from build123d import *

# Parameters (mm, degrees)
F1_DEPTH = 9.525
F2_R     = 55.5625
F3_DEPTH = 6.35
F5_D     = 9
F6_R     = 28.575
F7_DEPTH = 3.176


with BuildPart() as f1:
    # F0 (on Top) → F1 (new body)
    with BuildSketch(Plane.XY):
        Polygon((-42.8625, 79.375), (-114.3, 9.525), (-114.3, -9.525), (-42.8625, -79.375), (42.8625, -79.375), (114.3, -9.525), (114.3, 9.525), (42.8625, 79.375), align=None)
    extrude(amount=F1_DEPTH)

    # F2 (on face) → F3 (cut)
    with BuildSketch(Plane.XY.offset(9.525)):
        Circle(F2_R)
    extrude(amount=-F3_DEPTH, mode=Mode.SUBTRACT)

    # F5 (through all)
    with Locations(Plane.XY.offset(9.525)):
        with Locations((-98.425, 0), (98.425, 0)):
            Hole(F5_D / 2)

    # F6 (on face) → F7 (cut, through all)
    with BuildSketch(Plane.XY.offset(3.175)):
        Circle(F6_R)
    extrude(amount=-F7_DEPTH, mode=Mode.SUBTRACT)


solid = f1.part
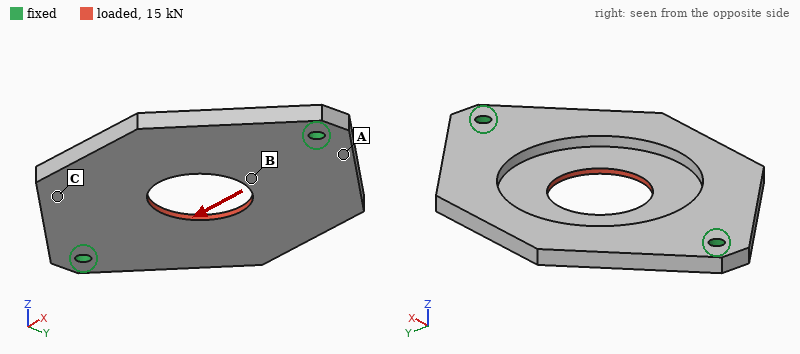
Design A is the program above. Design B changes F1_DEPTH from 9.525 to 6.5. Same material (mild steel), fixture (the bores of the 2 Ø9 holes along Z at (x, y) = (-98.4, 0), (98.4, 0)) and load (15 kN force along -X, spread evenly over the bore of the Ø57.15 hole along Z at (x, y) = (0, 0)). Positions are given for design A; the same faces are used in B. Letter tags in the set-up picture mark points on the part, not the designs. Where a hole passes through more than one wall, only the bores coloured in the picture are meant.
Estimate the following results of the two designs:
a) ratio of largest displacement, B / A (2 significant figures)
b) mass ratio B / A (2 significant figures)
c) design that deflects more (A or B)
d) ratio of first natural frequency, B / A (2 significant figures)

1.2
0.72
B
0.69
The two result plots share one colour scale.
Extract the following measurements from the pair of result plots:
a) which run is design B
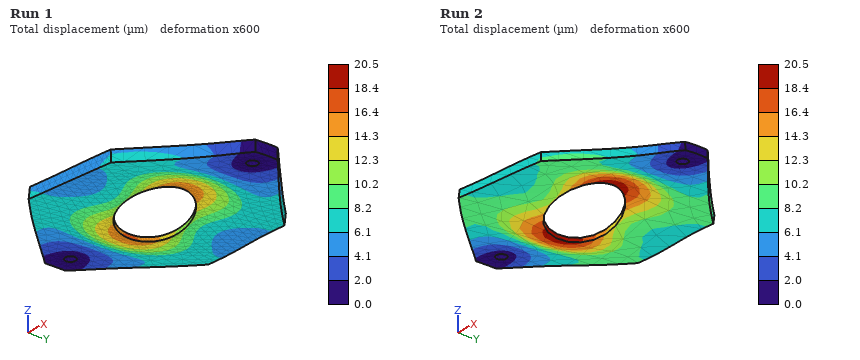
Run 2
